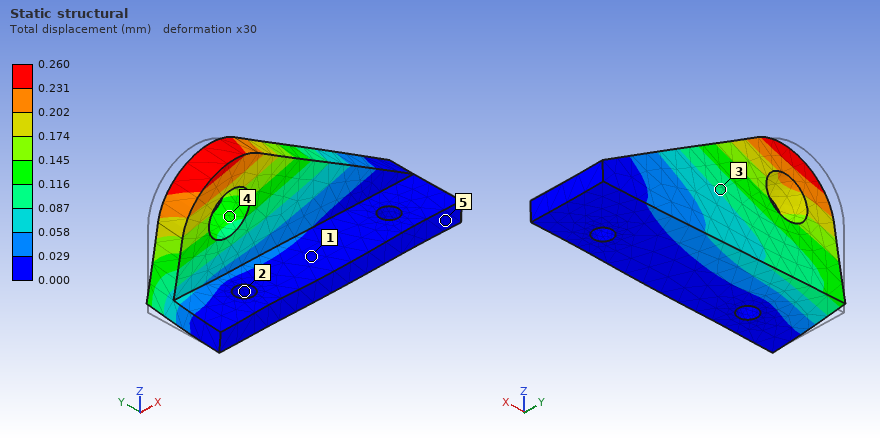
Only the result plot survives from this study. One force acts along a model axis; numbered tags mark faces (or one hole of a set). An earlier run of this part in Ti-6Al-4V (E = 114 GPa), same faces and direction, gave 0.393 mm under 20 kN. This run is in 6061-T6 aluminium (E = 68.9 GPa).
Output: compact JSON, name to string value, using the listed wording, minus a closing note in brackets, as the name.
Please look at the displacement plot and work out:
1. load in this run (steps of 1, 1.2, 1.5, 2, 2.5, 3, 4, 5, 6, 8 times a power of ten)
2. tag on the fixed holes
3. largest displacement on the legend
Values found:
{"load in this run": "8 kN", "tag on the fixed holes": "2", "largest displacement on the legend": "0.260 mm"}
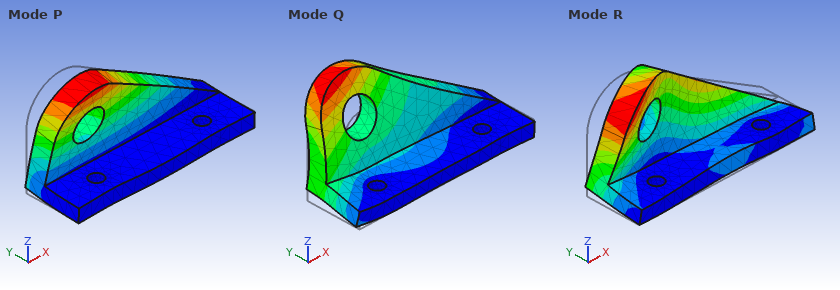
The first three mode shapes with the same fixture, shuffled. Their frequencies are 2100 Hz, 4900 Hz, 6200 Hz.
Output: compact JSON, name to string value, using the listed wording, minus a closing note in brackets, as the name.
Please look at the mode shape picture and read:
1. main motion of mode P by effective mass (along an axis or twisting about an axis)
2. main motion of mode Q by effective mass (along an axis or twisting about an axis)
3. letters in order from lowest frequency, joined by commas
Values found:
{"main motion of mode P by effective mass": "along Y", "main motion of mode Q by effective mass": "along Z", "letters in order from lowest frequency, joined by commas": "P, R, Q"}
